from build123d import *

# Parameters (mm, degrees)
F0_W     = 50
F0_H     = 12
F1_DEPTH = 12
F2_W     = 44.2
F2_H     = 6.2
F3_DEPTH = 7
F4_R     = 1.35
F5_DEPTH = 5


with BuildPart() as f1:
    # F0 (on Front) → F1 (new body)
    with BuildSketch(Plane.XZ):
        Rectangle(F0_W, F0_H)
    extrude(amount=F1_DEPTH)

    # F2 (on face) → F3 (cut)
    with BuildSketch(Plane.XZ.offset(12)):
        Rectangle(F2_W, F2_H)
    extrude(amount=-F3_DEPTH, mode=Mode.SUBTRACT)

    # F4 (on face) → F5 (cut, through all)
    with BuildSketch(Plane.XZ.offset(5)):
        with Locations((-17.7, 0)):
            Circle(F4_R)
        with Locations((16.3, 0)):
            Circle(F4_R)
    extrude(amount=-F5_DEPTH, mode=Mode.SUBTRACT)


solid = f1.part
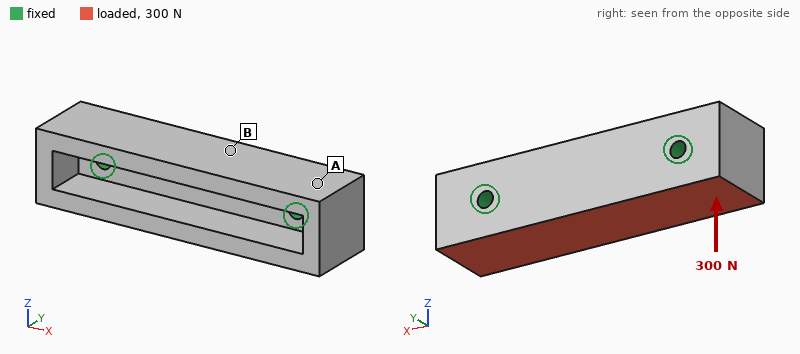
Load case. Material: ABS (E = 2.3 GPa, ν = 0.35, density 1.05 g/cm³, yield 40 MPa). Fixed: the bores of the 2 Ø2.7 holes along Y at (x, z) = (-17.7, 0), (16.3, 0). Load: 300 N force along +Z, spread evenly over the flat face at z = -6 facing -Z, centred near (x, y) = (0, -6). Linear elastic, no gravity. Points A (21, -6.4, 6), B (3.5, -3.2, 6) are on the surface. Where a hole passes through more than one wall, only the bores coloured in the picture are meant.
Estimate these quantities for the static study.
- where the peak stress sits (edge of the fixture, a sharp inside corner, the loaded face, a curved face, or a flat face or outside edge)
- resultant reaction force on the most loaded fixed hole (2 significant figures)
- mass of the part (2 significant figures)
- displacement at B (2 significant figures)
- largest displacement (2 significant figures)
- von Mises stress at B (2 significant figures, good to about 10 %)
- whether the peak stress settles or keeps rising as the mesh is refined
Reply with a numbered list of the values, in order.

1. edge of the fixture
2. 160 N
3. 5.5 g
4. 0.051 mm
5. 0.18 mm
6. 2.9 MPa
7. keeps rising
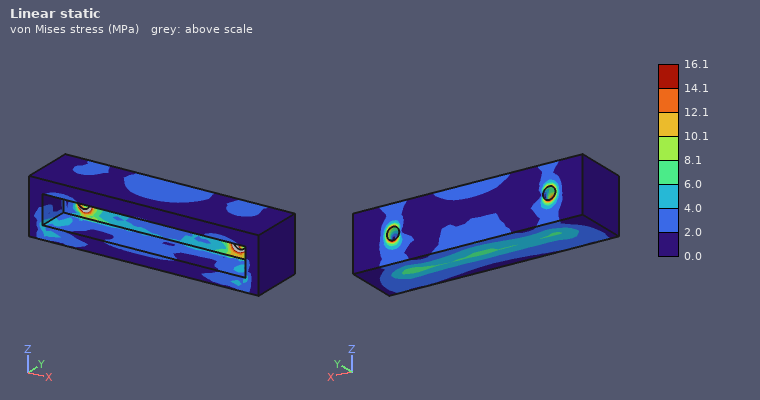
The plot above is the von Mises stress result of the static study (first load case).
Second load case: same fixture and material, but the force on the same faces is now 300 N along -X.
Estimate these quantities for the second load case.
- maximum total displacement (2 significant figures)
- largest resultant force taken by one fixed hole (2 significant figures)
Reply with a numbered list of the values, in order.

1. 37 µm
2. 160 N
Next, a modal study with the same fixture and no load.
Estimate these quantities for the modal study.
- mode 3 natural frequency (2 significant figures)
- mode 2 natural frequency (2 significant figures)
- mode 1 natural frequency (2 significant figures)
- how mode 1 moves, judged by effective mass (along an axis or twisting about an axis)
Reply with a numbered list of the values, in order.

1. 6600 Hz
2. 6500 Hz
3. 4600 Hz
4. along Z
